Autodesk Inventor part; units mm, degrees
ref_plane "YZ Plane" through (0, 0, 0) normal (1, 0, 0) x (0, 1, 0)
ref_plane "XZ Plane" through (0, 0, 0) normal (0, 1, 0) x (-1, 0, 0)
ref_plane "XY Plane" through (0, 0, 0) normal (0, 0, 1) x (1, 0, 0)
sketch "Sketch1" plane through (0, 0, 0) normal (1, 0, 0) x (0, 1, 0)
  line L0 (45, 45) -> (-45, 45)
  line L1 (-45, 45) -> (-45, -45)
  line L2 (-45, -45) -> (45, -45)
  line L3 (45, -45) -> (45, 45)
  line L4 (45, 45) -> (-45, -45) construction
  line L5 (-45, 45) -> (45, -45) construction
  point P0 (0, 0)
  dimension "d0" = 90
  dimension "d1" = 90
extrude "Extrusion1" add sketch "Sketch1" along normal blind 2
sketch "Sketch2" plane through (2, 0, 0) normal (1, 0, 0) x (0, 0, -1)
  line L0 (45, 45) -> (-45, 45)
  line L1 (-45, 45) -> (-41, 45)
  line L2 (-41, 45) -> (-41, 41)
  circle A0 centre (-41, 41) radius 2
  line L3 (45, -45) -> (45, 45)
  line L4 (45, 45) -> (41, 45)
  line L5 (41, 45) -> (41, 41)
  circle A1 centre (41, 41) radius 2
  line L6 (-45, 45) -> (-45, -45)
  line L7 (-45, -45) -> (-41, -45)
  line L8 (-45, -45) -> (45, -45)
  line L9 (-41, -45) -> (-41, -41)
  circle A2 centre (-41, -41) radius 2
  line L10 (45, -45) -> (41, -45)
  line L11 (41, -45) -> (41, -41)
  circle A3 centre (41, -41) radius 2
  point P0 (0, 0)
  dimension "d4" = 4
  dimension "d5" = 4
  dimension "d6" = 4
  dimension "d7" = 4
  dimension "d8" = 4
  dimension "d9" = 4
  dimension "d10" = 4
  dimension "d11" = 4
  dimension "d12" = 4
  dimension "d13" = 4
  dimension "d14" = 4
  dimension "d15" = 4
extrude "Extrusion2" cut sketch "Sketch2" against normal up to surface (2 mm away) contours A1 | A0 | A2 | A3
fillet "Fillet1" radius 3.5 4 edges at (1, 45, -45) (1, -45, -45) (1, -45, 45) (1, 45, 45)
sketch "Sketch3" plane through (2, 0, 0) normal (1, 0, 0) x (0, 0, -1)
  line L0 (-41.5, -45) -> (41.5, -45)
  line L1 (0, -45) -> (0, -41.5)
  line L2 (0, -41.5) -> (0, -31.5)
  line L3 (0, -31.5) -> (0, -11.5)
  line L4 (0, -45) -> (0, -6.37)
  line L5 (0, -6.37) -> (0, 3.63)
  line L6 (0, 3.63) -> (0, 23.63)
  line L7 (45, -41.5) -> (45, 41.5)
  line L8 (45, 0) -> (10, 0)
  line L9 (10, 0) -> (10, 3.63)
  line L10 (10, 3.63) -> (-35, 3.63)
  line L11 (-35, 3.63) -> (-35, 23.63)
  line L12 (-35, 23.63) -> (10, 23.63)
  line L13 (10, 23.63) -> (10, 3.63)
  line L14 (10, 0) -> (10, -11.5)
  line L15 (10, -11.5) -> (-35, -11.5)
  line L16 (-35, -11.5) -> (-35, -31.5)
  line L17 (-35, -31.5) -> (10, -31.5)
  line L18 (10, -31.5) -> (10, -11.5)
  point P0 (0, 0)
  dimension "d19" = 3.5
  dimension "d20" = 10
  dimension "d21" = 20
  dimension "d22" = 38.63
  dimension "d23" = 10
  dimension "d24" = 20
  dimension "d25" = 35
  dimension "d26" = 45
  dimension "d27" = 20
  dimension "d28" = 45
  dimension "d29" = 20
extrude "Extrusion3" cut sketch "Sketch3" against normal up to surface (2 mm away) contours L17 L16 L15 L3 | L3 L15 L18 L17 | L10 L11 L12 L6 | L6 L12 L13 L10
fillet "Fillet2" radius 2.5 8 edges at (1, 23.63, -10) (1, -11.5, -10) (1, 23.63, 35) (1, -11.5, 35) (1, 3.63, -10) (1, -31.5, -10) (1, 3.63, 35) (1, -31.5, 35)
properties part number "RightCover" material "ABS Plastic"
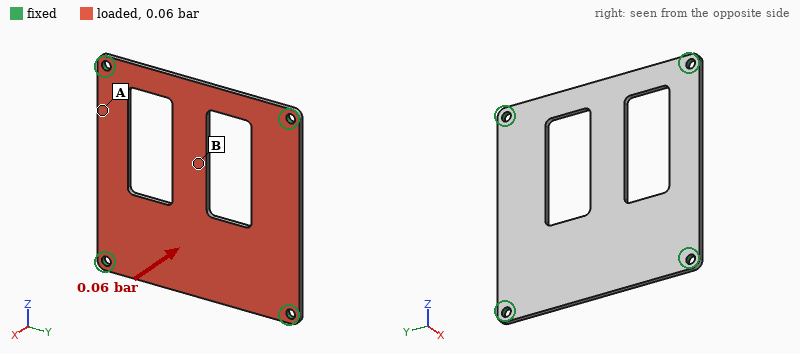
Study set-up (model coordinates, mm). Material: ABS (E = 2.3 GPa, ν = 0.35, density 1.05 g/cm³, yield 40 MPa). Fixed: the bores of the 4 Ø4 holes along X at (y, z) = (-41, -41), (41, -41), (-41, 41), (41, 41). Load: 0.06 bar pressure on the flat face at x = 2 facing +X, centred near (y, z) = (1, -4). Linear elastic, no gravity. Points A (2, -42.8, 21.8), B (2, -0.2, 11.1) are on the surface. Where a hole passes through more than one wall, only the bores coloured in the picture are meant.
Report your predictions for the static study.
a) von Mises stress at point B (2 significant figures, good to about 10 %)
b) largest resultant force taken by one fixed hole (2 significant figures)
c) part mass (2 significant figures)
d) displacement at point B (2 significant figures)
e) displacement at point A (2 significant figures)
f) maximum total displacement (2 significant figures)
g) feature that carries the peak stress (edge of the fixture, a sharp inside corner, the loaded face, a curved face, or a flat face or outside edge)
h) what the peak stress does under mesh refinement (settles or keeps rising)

3.5 MPa
11 N
13 g
1.4 mm
0.25 mm
1.5 mm
edge of the fixture
keeps rising
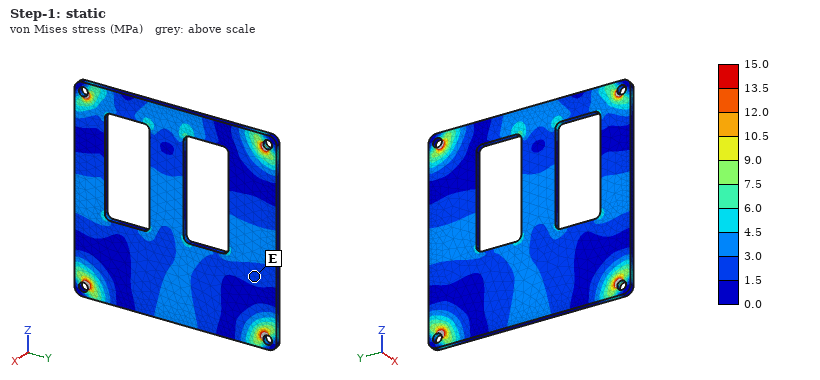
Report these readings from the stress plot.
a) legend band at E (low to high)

1.5 to 3.0 MPa
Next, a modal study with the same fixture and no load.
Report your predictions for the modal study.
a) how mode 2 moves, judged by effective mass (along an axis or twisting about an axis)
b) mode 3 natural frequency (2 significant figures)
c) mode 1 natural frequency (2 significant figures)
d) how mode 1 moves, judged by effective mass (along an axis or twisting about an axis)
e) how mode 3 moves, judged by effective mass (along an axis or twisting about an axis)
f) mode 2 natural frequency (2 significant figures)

twisting about Y
500 Hz
290 Hz
along X
twisting about Z
470 Hz
